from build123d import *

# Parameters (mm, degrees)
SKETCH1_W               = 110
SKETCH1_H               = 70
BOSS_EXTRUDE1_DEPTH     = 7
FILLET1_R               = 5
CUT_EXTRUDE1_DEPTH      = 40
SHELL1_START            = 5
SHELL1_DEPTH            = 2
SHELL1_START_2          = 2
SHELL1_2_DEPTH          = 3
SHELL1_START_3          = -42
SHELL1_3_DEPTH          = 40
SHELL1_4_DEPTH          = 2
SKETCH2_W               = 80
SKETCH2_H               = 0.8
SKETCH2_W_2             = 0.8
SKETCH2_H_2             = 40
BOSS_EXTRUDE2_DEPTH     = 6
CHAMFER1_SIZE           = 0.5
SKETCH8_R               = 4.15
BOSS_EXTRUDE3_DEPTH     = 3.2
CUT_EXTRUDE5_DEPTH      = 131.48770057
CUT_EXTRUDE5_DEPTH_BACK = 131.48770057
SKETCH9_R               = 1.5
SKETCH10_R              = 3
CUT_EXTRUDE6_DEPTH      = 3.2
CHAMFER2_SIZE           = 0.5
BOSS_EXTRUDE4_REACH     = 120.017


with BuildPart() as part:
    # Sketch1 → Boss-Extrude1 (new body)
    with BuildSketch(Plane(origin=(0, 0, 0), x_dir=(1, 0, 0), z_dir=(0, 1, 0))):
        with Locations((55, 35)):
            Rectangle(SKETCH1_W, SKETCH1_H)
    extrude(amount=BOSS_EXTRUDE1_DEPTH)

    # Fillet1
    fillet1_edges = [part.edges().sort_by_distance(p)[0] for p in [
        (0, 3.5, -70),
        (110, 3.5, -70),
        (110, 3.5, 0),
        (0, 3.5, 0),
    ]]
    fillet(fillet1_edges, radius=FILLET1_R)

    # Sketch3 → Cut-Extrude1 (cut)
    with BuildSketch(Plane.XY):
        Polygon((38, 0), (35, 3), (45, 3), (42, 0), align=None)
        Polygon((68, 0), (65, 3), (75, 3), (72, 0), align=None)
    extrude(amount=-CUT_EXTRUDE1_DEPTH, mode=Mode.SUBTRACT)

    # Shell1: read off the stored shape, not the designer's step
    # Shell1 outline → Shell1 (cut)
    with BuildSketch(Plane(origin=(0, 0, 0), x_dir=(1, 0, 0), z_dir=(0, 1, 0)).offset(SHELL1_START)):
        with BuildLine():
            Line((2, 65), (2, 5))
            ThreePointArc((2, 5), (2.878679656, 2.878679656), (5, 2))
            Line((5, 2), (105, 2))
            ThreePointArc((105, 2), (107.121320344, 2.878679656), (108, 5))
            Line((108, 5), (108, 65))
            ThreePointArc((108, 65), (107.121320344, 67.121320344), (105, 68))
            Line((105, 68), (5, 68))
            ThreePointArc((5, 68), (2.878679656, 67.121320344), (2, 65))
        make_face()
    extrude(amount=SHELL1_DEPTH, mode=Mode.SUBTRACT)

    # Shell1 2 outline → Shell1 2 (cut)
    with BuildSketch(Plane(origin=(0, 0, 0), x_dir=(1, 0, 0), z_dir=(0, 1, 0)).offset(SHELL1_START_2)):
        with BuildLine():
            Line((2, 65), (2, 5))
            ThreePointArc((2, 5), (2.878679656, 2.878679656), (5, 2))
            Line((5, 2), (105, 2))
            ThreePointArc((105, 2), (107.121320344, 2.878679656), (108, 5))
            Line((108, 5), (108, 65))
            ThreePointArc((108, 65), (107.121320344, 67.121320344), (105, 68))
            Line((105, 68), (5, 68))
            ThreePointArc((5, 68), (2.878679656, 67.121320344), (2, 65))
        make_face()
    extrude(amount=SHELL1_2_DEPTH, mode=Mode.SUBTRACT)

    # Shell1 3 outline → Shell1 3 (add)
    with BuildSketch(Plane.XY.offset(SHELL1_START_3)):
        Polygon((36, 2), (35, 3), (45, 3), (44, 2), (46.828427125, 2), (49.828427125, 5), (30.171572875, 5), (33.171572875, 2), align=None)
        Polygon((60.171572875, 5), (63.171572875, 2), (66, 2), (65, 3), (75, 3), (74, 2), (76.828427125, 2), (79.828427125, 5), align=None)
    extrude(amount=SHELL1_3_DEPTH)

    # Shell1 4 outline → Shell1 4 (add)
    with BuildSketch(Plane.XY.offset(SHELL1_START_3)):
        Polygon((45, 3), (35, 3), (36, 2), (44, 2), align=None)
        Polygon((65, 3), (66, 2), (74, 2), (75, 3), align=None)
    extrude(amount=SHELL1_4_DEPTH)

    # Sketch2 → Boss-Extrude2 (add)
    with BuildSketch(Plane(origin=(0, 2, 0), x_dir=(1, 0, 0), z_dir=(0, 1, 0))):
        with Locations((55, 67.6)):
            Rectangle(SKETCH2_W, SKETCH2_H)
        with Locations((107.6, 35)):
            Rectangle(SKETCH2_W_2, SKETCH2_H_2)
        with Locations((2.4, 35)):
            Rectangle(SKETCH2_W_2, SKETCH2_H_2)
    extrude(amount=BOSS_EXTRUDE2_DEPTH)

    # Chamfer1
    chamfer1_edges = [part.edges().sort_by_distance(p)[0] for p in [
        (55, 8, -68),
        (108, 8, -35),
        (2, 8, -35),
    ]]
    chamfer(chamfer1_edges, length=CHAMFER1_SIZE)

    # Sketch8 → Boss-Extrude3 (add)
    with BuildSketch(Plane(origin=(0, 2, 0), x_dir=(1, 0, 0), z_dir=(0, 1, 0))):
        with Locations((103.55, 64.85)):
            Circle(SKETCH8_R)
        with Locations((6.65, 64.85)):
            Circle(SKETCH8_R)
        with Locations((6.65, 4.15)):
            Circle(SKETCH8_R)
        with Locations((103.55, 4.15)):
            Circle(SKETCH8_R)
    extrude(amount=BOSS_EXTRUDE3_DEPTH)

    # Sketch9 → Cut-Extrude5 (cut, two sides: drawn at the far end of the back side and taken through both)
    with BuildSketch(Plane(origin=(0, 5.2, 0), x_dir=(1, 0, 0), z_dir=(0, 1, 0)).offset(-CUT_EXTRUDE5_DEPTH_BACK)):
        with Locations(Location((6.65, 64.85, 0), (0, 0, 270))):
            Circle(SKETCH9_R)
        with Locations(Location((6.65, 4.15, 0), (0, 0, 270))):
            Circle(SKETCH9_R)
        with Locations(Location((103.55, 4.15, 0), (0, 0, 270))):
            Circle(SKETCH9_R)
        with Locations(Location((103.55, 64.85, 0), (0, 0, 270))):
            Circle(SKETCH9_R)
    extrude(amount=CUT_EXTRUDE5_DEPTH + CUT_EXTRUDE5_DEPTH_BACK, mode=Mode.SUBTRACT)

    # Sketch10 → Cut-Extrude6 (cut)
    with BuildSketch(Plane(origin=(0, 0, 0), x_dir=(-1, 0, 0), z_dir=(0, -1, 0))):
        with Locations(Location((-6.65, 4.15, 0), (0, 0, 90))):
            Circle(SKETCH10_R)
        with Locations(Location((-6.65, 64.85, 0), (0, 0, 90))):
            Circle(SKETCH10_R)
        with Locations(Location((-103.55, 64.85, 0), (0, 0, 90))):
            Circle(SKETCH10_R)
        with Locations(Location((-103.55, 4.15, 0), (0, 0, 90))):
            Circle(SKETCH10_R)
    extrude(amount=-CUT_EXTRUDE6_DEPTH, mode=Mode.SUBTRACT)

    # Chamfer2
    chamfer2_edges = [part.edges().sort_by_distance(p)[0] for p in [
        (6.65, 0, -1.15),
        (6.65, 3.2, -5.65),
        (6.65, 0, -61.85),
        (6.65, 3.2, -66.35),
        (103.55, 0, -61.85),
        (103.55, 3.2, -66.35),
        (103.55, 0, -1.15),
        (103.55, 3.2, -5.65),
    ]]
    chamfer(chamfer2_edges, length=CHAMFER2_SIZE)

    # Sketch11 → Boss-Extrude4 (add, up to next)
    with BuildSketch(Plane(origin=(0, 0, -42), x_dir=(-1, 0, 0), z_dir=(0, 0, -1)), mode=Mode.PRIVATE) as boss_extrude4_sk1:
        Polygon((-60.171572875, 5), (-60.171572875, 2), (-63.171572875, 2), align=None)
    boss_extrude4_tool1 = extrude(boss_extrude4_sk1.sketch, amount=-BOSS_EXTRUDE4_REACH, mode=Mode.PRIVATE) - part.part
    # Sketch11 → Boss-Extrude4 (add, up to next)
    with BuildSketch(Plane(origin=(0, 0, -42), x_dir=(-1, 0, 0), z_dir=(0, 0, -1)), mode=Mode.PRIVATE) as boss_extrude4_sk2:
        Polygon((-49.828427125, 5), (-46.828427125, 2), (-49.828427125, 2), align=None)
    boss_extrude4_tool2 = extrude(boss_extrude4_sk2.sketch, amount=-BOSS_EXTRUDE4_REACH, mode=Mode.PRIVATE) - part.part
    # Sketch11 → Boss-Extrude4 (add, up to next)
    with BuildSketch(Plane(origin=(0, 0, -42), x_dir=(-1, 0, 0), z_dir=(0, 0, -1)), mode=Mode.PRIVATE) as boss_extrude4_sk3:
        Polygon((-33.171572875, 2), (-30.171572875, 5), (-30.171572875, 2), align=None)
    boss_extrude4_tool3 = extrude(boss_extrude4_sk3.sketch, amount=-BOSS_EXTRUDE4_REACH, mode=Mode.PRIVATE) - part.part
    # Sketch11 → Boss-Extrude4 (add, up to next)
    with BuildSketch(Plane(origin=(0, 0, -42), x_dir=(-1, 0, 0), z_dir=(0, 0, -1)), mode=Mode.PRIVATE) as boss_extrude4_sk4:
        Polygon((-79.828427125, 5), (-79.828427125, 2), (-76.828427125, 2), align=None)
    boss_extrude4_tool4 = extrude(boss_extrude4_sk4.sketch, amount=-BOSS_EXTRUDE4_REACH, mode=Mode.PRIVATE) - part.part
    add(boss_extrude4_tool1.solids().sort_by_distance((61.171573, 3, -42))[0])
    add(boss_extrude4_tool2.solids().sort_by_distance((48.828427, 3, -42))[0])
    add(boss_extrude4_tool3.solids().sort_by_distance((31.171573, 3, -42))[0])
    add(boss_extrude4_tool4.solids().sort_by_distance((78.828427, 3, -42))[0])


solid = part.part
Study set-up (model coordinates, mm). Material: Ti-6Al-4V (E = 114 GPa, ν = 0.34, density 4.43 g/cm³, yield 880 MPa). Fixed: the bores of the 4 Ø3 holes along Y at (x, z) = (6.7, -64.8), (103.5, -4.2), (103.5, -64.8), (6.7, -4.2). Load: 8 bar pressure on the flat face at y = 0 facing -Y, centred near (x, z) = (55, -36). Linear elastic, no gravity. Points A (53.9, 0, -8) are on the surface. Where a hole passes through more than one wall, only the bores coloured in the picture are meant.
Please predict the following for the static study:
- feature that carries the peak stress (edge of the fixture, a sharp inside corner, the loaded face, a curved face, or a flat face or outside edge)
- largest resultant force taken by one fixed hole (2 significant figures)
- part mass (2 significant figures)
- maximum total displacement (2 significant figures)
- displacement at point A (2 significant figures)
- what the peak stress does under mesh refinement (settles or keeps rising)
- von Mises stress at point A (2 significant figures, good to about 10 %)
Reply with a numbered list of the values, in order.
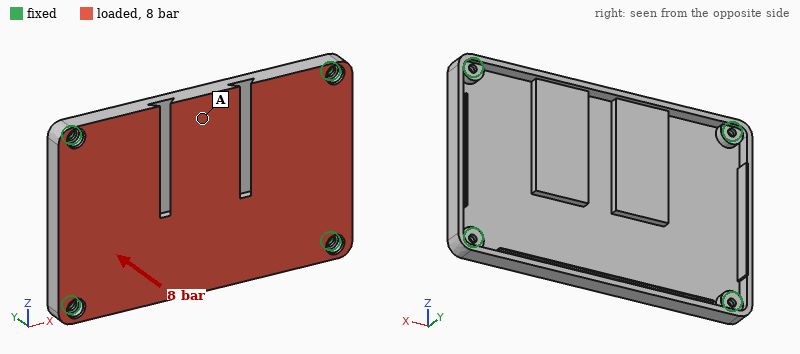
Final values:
1. edge of the fixture
2. 3.2 kN
3. 100 g
4. 1.2 mm
5. 0.96 mm
6. keeps rising
7. 140 MPa
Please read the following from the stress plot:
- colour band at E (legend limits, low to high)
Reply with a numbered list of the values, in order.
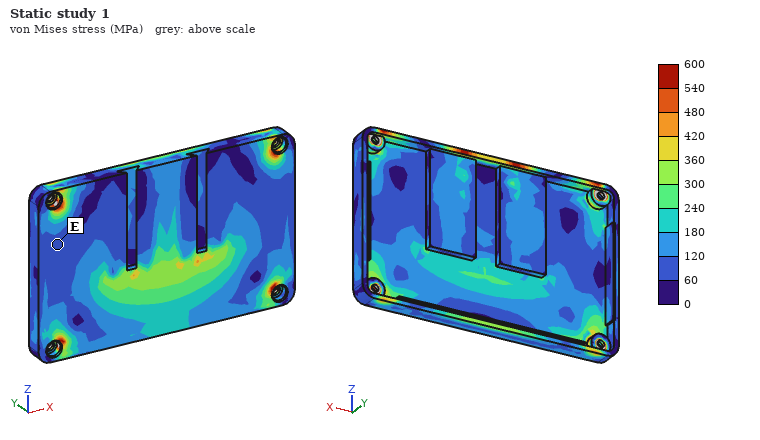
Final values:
1. 60 to 120 MPa
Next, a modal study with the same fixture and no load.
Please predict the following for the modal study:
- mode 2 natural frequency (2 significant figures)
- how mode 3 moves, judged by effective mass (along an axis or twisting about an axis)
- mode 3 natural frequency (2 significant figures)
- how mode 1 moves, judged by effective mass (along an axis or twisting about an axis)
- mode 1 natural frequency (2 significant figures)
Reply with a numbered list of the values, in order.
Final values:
1. 2300 Hz
2. twisting about Z
3. 3100 Hz
4. along Y
5. 1300 Hz
